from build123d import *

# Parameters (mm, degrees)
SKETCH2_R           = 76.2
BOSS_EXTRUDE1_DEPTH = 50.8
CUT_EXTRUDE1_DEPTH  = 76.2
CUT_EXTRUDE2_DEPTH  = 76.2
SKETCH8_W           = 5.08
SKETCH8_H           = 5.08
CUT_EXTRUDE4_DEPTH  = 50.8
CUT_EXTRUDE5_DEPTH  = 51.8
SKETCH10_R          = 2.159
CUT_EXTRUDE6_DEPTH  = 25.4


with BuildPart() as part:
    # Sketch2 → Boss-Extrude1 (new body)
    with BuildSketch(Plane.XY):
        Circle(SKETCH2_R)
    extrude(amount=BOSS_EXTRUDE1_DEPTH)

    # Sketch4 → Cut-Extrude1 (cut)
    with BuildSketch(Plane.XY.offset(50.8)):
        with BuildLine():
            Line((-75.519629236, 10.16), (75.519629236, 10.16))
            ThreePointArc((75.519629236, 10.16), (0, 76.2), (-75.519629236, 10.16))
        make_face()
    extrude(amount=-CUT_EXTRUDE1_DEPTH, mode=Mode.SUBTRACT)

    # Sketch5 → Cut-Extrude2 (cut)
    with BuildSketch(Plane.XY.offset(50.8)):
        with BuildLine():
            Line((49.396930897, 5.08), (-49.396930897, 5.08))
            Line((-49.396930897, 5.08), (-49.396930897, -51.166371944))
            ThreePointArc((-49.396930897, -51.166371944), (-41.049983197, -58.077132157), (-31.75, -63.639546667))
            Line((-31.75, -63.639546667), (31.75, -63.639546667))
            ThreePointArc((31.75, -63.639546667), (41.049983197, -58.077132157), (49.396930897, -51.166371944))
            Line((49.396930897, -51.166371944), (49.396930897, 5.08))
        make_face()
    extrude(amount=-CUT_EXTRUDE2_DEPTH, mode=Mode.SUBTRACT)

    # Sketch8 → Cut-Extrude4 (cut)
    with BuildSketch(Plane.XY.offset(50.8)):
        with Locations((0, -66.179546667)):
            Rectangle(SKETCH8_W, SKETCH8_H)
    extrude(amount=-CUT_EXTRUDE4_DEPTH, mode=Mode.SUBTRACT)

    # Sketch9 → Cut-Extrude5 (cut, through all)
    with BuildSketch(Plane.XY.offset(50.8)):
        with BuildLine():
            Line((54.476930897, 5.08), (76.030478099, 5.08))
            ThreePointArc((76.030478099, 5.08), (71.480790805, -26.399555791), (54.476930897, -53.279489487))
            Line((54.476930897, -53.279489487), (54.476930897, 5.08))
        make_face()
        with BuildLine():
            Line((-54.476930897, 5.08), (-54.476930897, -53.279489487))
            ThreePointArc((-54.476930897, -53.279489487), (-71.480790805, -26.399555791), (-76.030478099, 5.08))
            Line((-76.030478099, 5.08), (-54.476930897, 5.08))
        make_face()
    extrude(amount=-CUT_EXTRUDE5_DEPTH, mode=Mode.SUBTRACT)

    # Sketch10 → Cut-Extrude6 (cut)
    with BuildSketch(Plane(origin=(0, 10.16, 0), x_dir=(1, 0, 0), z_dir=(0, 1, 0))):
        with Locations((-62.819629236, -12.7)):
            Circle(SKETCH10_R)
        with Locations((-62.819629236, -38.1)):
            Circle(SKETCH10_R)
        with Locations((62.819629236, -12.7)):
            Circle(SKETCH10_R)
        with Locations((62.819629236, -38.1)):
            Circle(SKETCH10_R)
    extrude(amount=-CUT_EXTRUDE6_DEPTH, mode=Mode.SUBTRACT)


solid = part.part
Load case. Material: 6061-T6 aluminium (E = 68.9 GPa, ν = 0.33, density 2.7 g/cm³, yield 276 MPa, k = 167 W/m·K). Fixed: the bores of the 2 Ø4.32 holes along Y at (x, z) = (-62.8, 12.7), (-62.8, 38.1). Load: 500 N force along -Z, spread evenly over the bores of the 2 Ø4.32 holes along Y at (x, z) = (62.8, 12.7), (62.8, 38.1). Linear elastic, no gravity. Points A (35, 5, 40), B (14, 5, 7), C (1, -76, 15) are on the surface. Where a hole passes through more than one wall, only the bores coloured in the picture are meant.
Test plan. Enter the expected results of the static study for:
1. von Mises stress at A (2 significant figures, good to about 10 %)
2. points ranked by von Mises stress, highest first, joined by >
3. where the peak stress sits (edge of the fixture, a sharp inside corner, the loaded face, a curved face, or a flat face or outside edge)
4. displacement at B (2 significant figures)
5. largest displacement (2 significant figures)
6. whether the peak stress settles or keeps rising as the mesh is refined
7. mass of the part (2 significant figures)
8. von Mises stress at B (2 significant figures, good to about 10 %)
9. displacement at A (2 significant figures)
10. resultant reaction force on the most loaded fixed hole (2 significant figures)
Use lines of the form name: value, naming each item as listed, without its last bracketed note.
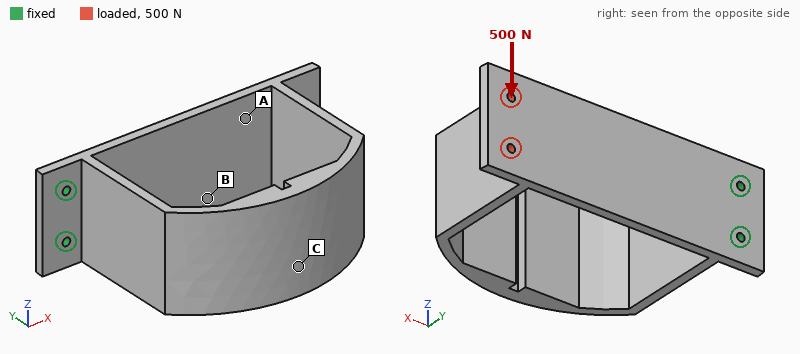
von Mises stress at A: 4.7 MPa
points ranked by von Mises stress, highest first, joined by >: B > A > C
where the peak stress sits: edge of the fixture
displacement at B: 0.063 mm
largest displacement: 0.14 mm
whether the peak stress settles or keeps rising as the mesh is refined: keeps rising
mass of the part: 310 g
von Mises stress at B: 8.1 MPa
displacement at A: 0.086 mm
resultant reaction force on the most loaded fixed hole: 2.3 kN
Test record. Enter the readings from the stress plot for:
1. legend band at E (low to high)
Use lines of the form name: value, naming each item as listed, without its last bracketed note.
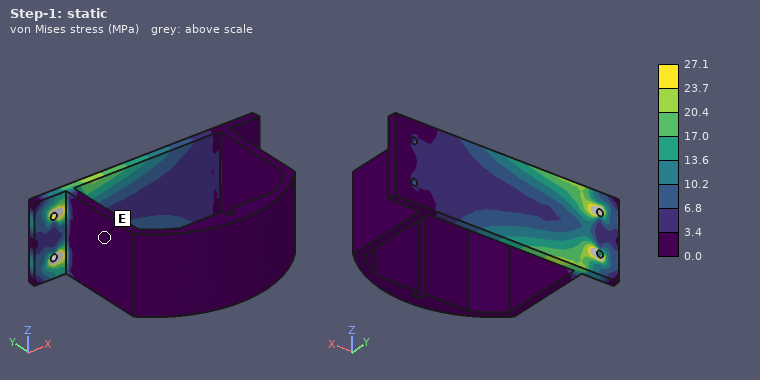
legend band at E: 0.0 to 3.4 MPa
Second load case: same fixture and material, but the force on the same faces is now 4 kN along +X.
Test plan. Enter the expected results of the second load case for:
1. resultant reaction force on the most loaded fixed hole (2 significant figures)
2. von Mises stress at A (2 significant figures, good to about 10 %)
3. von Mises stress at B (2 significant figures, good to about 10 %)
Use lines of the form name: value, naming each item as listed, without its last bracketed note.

resultant reaction force on the most loaded fixed hole: 2.0 kN
von Mises stress at A: 15 MPa
von Mises stress at B: 15 MPa
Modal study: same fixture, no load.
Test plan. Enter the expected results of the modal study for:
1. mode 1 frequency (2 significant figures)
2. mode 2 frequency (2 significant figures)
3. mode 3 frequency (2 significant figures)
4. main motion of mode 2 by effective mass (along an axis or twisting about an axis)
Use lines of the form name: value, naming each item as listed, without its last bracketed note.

mode 1 frequency: 140 Hz
mode 2 frequency: 520 Hz
mode 3 frequency: 660 Hz
main motion of mode 2 by effective mass: along Z
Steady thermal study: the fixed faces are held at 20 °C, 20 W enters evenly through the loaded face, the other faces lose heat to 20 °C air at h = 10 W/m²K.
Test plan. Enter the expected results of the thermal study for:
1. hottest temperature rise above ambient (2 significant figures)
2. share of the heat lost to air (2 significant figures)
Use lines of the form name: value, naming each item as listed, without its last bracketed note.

hottest temperature rise above ambient: 36 K
share of the heat lost to air: 33 %
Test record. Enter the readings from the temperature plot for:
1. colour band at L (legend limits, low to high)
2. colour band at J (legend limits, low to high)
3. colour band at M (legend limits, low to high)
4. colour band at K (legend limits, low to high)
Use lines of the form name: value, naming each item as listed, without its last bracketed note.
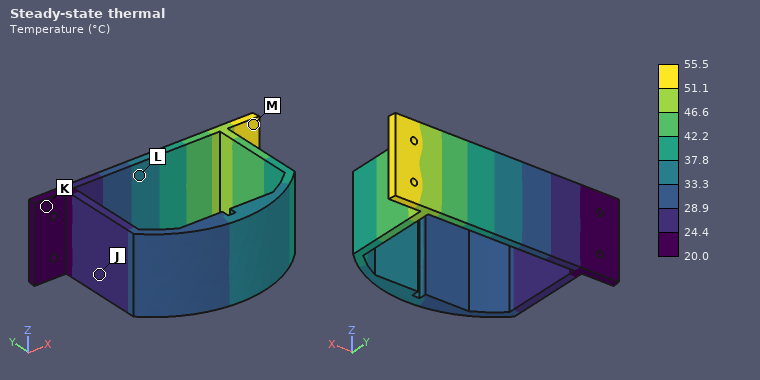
colour band at L: 33.3 to 37.8 °C
colour band at J: 24.4 to 28.9 °C
colour band at M: 51.1 to 55.5 °C
colour band at K: 20.0 to 24.4 °C
